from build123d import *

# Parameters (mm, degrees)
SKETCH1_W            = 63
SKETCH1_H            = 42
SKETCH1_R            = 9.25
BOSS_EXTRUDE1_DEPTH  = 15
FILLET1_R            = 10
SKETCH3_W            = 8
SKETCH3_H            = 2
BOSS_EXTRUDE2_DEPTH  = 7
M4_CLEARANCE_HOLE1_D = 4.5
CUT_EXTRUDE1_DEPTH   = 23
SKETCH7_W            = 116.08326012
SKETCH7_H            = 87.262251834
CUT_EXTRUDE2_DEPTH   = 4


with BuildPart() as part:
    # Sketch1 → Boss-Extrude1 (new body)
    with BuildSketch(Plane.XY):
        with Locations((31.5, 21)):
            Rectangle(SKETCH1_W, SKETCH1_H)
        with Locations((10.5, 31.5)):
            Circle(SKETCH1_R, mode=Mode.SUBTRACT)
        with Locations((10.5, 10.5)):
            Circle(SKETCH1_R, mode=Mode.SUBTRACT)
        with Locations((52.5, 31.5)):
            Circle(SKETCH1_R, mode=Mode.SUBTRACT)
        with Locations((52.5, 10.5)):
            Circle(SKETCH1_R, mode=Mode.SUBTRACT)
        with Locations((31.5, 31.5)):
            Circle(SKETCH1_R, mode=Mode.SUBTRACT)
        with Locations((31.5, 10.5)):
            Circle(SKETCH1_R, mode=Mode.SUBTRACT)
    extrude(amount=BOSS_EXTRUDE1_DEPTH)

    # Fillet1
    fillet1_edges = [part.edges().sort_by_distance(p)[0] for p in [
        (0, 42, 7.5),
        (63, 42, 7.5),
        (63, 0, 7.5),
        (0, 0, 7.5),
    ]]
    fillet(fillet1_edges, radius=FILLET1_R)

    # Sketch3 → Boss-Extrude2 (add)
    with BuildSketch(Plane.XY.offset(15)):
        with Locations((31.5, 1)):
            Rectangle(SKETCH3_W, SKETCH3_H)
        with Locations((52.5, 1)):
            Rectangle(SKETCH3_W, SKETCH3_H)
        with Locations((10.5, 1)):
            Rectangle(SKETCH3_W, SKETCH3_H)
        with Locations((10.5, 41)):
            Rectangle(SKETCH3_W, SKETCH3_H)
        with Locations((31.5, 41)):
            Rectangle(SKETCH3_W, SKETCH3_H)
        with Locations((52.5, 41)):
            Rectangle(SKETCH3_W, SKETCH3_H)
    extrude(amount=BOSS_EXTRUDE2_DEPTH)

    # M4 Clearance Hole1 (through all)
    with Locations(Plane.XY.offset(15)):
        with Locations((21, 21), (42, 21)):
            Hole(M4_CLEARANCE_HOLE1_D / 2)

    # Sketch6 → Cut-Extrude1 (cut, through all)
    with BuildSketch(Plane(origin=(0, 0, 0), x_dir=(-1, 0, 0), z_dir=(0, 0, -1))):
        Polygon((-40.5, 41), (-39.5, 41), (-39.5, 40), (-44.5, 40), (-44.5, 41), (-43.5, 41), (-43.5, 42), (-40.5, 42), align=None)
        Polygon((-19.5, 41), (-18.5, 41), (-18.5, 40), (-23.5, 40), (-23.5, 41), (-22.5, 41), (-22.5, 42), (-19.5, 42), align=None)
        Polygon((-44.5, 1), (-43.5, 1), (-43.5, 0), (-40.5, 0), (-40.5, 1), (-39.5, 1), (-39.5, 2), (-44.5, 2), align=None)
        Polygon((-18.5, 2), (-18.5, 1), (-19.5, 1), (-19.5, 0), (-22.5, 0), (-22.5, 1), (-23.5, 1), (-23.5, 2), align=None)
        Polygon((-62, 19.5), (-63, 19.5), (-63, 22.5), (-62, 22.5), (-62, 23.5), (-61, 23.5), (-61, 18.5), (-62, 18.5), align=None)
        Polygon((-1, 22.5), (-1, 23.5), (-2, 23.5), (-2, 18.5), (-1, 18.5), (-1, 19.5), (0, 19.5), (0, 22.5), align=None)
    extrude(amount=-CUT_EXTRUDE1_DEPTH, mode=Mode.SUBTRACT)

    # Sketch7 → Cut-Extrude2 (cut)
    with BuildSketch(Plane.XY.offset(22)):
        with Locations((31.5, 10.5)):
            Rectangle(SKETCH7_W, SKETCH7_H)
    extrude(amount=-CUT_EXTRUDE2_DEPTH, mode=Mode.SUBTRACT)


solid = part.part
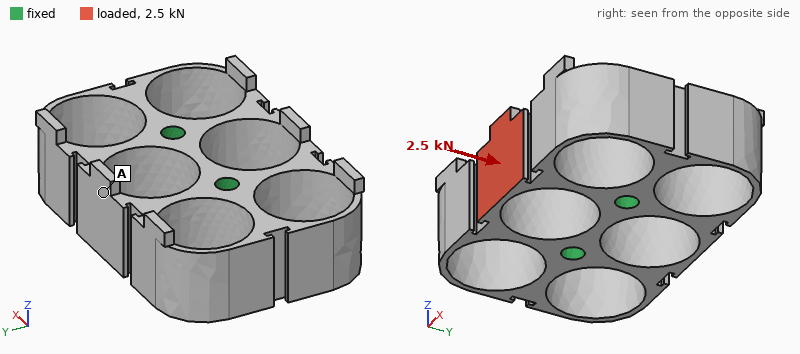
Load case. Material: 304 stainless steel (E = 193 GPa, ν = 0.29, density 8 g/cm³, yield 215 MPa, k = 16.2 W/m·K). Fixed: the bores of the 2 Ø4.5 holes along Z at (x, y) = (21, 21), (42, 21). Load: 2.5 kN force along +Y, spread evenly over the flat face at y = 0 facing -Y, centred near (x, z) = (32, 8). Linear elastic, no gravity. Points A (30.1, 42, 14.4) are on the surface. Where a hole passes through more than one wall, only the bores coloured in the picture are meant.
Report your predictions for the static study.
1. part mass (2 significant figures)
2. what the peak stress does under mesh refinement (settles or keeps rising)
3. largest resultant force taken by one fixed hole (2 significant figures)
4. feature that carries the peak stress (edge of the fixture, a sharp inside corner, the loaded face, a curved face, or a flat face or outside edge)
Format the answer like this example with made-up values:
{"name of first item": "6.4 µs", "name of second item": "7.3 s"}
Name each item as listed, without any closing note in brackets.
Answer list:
{"part mass": "110 g", "what the peak stress does under mesh refinement": "keeps rising", "largest resultant force taken by one fixed hole": "1.4 kN", "feature that carries the peak stress": "a sharp inside corner"}
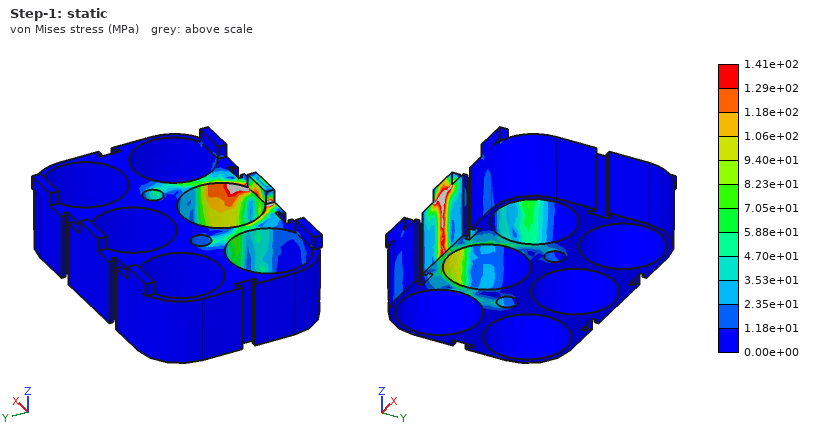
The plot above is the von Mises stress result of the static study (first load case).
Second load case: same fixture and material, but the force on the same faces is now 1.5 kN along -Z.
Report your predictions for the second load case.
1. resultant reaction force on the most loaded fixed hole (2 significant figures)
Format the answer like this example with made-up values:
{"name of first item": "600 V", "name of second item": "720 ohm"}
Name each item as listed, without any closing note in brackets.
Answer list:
{"resultant reaction force on the most loaded fixed hole": "750 N"}
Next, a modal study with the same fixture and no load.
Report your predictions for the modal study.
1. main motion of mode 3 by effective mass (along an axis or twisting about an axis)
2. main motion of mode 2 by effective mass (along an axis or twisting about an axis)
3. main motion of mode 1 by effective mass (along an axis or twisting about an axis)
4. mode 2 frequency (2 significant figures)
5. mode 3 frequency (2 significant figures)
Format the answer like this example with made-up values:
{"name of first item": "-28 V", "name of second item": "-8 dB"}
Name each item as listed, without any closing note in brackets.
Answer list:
{"main motion of mode 3 by effective mass": "along X", "main motion of mode 2 by effective mass": "along Y", "main motion of mode 1 by effective mass": "twisting about Z", "mode 2 frequency": "7500 Hz", "mode 3 frequency": "8800 Hz"}
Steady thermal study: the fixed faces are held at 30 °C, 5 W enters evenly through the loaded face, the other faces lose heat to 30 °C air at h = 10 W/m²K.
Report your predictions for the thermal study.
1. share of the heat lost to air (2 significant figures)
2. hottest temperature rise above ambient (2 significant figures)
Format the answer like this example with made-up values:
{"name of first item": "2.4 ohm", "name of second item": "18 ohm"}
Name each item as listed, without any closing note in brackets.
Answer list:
{"share of the heat lost to air": "18 %", "hottest temperature rise above ambient": "60 K"}
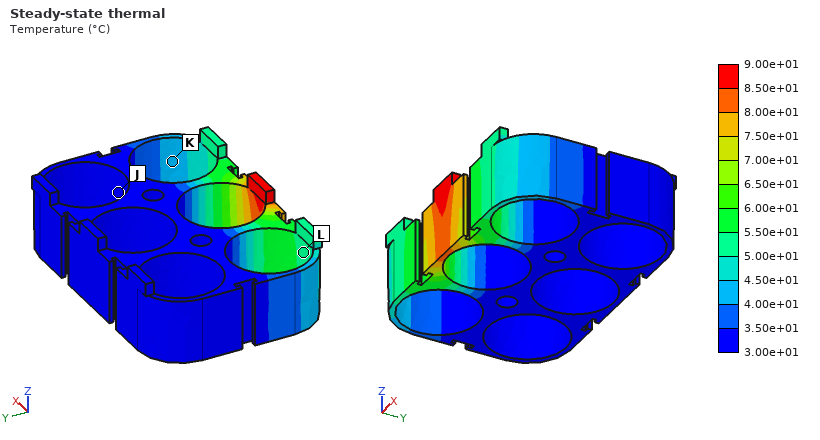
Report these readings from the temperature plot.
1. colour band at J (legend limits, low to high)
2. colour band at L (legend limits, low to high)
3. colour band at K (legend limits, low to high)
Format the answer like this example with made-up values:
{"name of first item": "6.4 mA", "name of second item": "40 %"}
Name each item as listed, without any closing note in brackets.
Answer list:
{"colour band at J": "3.00e+01 to 3.50e+01 °C", "colour band at L": "5.00e+01 to 5.50e+01 °C", "colour band at K": "4.00e+01 to 4.50e+01 °C"}
